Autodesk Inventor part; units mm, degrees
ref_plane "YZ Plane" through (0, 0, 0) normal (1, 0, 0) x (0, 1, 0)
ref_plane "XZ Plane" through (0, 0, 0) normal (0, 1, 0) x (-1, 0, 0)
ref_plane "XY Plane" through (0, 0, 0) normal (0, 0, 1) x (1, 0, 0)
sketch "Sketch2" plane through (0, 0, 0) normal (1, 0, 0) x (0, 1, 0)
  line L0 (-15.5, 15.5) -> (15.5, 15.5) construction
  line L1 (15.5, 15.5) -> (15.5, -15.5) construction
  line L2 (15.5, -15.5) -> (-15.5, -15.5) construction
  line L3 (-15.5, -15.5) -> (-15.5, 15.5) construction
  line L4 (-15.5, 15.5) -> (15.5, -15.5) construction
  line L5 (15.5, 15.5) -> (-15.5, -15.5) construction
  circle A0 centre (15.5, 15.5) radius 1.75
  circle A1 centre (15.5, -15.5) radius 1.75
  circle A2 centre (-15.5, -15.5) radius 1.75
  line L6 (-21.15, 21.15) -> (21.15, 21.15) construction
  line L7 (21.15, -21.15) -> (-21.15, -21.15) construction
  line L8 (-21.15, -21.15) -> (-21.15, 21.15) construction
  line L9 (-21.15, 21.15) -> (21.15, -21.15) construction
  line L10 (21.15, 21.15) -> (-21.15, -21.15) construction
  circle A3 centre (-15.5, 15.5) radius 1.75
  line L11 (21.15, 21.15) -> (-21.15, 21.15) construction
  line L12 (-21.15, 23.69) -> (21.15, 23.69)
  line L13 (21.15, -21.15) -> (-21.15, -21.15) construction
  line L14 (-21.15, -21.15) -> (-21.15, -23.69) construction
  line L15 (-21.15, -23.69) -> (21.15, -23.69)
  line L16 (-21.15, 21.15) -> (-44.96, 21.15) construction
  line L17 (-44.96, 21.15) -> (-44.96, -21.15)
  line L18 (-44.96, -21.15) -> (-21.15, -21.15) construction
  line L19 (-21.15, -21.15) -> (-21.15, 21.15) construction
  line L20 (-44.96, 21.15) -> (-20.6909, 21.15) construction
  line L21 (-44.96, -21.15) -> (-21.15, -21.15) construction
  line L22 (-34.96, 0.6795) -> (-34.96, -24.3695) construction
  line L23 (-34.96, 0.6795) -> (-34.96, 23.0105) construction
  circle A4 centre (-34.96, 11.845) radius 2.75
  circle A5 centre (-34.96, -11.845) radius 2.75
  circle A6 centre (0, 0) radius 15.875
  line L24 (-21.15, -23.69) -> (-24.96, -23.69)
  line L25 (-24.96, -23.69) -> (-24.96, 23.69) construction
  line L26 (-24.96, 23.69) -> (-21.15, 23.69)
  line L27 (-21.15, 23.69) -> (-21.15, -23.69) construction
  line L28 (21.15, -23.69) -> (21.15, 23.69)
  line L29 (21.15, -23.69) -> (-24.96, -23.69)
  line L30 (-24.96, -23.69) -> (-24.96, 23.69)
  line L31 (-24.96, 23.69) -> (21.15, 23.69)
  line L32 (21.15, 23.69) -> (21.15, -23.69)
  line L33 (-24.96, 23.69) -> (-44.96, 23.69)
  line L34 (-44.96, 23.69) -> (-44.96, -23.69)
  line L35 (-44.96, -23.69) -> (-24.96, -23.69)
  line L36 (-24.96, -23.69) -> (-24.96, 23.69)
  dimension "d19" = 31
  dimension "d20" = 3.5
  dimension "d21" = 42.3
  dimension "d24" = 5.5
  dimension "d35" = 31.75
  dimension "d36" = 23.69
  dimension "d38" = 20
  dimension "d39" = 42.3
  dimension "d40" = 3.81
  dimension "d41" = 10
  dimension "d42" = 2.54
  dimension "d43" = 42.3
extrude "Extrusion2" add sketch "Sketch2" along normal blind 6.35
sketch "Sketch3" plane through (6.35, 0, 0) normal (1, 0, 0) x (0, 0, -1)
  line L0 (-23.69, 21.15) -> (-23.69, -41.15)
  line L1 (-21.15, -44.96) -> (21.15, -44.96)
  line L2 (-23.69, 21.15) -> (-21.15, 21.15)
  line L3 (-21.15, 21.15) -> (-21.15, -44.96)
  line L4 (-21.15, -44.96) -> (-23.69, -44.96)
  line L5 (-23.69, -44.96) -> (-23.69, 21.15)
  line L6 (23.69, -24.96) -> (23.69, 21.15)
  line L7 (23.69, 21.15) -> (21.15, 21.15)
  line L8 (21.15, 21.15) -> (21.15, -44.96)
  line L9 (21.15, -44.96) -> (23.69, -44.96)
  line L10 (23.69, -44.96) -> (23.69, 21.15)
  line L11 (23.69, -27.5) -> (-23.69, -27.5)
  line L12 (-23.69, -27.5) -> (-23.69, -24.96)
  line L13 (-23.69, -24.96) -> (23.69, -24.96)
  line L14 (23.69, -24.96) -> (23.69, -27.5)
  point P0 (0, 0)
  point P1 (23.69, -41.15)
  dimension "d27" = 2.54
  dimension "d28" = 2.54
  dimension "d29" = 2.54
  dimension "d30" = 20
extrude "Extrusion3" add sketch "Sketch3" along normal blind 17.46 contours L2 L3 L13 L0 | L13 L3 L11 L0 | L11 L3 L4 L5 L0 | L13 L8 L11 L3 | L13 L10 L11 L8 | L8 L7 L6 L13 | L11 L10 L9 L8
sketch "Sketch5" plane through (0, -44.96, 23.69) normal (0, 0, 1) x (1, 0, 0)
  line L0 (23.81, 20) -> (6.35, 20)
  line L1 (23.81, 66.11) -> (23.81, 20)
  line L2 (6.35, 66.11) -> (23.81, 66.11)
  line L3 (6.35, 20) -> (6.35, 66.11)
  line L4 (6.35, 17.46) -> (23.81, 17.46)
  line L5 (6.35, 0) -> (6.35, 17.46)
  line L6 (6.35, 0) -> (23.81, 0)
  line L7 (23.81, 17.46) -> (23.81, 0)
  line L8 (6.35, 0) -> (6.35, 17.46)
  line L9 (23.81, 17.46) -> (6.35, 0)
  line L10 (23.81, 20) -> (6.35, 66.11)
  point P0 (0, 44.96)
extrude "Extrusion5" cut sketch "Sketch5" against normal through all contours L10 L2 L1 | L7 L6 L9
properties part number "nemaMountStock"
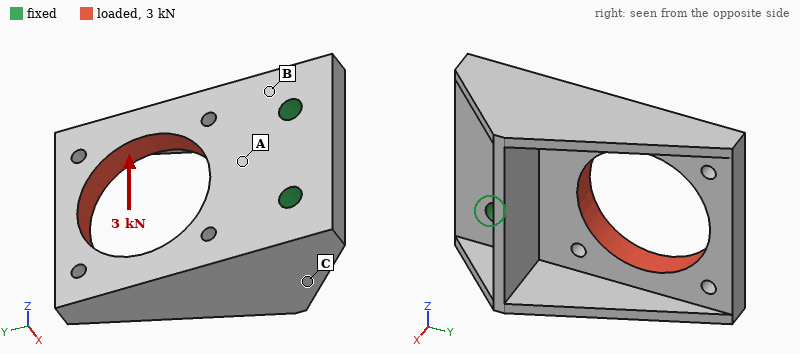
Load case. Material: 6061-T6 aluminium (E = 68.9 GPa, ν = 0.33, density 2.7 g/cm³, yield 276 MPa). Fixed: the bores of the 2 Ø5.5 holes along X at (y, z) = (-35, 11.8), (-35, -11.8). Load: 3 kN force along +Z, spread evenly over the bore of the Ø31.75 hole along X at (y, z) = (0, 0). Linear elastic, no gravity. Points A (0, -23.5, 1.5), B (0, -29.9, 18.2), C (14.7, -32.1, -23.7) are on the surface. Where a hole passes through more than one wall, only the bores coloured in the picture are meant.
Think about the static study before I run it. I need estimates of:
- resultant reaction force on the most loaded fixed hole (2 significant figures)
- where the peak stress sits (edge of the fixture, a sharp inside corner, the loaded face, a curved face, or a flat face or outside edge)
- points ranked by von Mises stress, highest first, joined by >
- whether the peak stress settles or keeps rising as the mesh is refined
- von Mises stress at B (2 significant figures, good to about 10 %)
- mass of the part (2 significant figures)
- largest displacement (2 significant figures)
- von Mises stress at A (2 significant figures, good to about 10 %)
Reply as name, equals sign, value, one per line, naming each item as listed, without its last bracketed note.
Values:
resultant reaction force on the most loaded fixed hole = 3.9 kN
where the peak stress sits = edge of the fixture
points ranked by von Mises stress, highest first, joined by > = A > B > C
whether the peak stress settles or keeps rising as the mesh is refined = keeps rising
von Mises stress at B = 27 MPa
mass of the part = 52 g
largest displacement = 0.15 mm
von Mises stress at A = 54 MPa
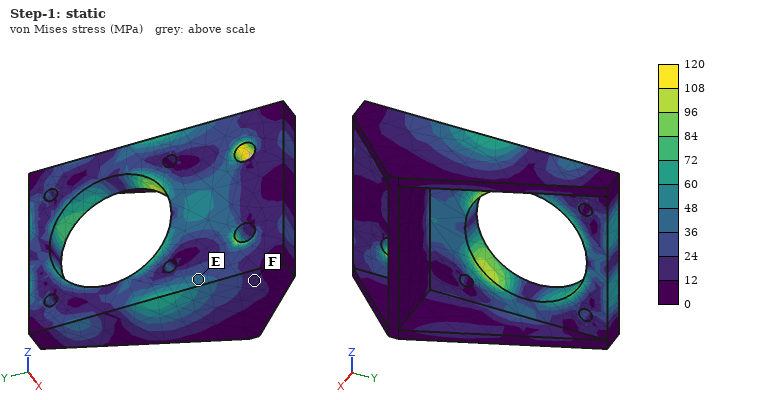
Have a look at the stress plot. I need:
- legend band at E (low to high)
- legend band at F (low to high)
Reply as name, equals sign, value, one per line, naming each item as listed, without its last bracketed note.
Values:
legend band at E = 36 to 48 MPa
legend band at F = 12 to 24 MPa
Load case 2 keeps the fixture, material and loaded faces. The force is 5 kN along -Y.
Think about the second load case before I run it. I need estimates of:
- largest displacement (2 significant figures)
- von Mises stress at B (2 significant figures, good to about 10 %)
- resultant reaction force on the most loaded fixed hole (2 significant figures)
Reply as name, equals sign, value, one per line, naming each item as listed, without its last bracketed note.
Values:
largest displacement = 61 µm
von Mises stress at B = 27 MPa
resultant reaction force on the most loaded fixed hole = 2.5 kN
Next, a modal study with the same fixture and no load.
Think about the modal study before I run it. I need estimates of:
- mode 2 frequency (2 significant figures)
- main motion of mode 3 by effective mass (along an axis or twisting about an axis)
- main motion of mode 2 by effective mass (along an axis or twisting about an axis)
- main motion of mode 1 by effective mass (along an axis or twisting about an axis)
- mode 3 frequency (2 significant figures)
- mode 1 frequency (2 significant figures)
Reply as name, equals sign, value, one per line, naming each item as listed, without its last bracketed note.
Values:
mode 2 frequency = 3700 Hz
main motion of mode 3 by effective mass = along Z
main motion of mode 2 by effective mass = twisting about Y
main motion of mode 1 by effective mass = along X
mode 3 frequency = 5600 Hz
mode 1 frequency = 2600 Hz
